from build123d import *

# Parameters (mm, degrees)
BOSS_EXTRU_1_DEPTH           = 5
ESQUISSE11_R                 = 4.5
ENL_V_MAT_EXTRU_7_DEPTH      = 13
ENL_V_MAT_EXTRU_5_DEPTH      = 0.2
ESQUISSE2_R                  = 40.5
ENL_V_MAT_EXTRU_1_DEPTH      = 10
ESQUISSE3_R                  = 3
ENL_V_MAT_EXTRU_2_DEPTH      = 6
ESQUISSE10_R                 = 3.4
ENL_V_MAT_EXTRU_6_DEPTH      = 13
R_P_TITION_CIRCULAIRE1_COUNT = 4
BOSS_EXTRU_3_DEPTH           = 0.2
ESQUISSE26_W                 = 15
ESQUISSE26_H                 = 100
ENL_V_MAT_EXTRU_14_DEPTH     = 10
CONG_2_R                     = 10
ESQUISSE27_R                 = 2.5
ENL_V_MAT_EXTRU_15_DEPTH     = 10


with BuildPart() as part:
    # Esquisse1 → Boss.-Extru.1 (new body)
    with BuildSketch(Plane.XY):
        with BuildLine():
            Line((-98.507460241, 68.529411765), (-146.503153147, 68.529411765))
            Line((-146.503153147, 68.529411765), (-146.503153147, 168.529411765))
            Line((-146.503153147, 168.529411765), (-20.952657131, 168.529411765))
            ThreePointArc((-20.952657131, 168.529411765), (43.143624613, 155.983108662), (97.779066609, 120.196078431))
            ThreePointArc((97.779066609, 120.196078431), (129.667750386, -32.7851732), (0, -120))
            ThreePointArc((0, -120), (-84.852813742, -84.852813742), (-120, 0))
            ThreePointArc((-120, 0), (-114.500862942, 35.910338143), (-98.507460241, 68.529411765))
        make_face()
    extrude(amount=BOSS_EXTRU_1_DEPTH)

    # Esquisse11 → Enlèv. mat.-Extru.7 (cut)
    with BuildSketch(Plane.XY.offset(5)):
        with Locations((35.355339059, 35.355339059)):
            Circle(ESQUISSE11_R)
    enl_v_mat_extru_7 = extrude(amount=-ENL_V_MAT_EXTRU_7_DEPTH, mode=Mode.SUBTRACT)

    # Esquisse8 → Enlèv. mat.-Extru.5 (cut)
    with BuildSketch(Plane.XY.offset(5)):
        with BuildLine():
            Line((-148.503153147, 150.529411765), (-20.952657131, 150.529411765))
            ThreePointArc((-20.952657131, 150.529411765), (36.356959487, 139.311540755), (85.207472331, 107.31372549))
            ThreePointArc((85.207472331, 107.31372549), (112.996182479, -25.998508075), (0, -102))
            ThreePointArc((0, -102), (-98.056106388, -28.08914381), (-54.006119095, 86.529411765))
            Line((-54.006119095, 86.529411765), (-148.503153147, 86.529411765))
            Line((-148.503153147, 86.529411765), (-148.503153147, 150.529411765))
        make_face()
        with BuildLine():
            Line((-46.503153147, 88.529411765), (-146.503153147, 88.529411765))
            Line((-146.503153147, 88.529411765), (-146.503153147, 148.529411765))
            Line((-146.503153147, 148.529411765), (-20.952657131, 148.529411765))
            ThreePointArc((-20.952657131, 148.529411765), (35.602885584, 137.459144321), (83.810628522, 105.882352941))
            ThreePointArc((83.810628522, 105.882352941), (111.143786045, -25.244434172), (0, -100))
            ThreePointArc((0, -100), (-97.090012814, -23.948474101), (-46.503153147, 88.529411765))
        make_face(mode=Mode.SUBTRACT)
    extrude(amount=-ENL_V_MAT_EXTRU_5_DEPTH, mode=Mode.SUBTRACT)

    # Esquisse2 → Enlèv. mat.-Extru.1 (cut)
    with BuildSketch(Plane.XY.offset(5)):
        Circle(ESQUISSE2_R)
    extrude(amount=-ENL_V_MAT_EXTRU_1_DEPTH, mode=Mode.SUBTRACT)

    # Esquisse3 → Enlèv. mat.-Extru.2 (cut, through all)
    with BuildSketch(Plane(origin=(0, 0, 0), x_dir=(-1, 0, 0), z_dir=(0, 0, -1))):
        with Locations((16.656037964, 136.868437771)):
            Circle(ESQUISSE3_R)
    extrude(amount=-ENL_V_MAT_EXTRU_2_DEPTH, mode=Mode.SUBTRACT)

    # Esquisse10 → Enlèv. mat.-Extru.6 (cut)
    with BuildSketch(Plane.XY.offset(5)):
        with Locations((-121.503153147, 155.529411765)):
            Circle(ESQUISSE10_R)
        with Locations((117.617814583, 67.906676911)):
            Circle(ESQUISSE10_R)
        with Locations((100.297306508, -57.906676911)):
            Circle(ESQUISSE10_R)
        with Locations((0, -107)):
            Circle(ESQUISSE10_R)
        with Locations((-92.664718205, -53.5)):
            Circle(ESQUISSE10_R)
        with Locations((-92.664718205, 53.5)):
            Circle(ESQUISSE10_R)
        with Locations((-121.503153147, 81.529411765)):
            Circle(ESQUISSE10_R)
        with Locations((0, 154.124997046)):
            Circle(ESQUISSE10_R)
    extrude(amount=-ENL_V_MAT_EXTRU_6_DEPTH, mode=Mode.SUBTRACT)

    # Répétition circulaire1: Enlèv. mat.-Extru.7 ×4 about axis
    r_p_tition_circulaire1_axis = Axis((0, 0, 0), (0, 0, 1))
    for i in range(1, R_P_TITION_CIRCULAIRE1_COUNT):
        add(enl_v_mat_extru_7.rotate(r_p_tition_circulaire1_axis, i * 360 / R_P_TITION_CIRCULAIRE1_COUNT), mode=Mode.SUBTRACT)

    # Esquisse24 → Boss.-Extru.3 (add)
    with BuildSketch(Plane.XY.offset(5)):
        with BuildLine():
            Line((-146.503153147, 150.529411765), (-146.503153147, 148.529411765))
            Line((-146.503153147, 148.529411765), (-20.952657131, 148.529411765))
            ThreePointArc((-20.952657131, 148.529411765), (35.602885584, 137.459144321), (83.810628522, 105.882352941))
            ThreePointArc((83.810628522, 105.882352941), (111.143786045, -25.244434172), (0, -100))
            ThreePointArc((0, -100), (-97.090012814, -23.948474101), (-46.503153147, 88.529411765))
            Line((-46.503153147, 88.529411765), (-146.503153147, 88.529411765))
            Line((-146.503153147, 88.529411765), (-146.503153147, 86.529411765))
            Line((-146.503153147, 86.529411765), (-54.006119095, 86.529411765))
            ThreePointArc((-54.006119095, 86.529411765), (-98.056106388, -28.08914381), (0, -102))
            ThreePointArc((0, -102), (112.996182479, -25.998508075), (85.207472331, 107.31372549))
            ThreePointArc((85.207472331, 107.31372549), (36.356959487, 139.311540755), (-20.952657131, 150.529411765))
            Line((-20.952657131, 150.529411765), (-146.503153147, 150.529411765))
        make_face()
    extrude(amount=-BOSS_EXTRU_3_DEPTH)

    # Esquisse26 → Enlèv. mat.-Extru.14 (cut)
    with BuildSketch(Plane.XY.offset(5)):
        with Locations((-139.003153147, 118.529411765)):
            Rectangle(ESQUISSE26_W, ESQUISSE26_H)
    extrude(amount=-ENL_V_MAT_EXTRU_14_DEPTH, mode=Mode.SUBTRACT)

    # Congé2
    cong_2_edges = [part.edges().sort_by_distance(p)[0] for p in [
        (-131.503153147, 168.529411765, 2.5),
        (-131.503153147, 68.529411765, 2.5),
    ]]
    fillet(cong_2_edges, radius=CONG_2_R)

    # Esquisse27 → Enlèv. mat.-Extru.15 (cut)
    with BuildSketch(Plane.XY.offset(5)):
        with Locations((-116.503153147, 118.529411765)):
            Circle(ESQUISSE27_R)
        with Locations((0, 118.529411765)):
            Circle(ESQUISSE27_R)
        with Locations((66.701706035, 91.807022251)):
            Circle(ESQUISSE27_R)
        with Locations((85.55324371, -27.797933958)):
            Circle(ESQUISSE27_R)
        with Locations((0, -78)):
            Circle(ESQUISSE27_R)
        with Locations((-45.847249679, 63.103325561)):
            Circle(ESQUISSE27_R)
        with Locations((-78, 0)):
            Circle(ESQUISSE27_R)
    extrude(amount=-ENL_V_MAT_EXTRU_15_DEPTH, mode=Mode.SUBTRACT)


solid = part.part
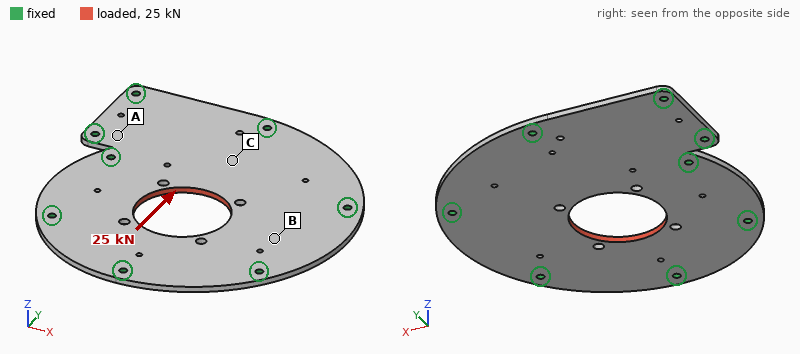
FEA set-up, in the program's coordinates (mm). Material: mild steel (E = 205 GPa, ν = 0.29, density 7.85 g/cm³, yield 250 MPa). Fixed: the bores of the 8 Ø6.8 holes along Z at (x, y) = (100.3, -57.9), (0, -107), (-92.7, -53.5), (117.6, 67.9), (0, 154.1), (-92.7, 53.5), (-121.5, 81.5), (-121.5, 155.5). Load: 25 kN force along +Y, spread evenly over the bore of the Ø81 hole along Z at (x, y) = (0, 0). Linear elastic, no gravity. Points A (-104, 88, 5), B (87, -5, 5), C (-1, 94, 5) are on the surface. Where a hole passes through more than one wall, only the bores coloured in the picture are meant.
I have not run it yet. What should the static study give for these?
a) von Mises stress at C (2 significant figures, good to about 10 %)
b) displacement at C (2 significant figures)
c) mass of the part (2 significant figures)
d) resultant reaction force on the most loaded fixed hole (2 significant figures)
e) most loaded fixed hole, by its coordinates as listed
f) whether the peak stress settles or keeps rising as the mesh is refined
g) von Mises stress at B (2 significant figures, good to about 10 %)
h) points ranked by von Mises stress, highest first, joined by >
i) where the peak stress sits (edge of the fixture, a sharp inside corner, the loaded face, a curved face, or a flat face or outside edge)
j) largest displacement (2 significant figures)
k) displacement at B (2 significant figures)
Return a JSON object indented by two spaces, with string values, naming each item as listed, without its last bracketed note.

{
  "von Mises stress at C": "17 MPa",
  "displacement at C": "6.5 µm",
  "mass of the part": "2.3 kg",
  "resultant reaction force on the most loaded fixed hole": "6.0 kN",
  "most loaded fixed hole, by its coordinates as listed": "(0, -107)",
  "whether the peak stress settles or keeps rising as the mesh is refined": "keeps rising",
  "von Mises stress at B": "9.5 MPa",
  "points ranked by von Mises stress, highest first, joined by >": "C > B > A",
  "where the peak stress sits": "edge of the fixture",
  "largest displacement": "12 µm",
  "displacement at B": "3.8 µm"
}
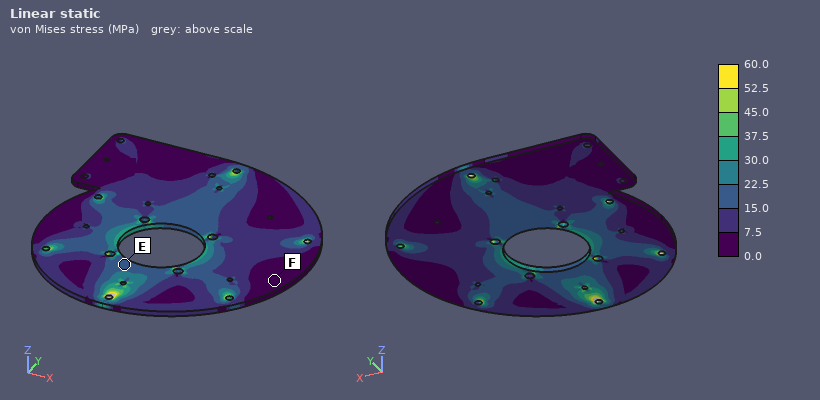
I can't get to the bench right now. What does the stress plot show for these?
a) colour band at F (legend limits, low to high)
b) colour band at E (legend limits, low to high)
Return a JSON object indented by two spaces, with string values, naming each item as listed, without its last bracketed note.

{
  "colour band at F": "0.0 to 7.5 MPa",
  "colour band at E": "15.0 to 22.5 MPa"
}
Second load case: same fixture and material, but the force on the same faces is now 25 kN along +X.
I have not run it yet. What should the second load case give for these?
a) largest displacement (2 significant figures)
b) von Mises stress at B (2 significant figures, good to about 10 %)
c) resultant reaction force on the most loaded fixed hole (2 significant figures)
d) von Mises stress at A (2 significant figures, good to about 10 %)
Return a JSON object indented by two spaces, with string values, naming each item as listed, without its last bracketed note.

{
  "largest displacement": "12 µm",
  "von Mises stress at B": "8.4 MPa",
  "resultant reaction force on the most loaded fixed hole": "5.4 kN",
  "von Mises stress at A": "7.8 MPa"
}
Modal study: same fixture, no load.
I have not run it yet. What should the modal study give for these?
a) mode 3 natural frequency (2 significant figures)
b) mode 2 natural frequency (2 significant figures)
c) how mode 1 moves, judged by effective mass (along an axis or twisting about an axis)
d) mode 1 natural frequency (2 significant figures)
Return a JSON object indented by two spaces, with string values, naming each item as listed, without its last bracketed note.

{
  "mode 3 natural frequency": "1300 Hz",
  "mode 2 natural frequency": "1200 Hz",
  "how mode 1 moves, judged by effective mass": "along Z",
  "mode 1 natural frequency": "740 Hz"
}
